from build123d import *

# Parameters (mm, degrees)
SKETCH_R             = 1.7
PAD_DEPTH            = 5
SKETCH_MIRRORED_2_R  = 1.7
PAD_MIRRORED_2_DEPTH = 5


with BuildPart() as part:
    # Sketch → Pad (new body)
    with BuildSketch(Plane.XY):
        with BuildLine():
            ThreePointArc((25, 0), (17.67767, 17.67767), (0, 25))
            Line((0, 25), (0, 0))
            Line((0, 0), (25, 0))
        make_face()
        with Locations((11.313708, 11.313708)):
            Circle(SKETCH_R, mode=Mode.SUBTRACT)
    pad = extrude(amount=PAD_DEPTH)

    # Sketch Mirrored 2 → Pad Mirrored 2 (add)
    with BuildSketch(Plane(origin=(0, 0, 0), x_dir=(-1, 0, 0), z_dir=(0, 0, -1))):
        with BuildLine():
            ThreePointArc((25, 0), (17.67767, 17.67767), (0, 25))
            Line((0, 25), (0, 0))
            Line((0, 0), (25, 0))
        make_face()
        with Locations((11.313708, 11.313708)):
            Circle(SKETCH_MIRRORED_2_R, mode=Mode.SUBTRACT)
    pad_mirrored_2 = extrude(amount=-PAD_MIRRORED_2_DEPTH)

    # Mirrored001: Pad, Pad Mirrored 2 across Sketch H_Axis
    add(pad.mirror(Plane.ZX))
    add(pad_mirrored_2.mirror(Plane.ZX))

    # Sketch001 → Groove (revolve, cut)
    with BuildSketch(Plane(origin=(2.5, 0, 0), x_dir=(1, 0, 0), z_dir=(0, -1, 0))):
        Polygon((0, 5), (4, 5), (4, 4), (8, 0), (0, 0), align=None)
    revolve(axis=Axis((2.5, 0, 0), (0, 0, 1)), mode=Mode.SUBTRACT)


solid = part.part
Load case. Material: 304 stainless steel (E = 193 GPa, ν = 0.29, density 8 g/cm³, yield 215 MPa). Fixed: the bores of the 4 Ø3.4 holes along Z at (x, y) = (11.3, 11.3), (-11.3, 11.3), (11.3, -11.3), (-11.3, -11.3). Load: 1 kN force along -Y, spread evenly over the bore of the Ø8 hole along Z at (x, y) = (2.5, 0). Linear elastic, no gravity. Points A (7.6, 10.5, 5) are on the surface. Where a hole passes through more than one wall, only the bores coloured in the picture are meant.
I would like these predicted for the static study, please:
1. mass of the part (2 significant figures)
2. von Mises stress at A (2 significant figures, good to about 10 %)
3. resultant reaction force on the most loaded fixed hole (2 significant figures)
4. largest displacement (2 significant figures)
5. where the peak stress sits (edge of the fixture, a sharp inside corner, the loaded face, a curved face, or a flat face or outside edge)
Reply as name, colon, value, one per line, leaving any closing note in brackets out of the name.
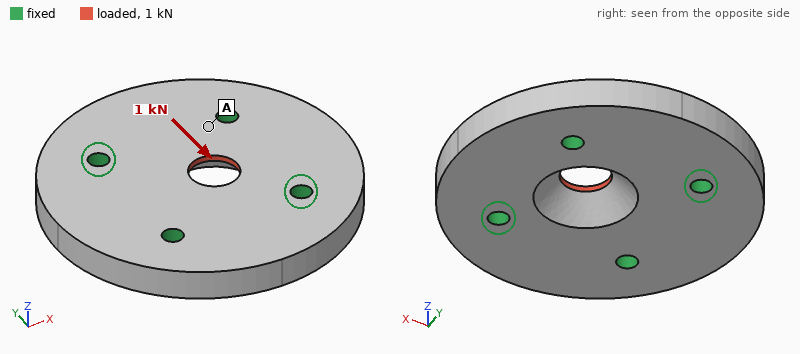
mass of the part: 73 g
von Mises stress at A: 7.8 MPa
resultant reaction force on the most loaded fixed hole: 300 N
largest displacement: 1.4 µm
where the peak stress sits: the loaded face
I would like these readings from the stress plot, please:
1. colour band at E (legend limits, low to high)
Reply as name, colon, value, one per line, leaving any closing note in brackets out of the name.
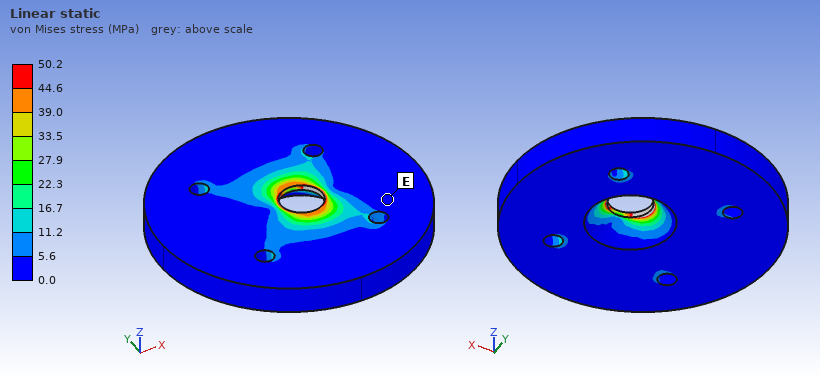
colour band at E: 0.0 to 5.6 MPa
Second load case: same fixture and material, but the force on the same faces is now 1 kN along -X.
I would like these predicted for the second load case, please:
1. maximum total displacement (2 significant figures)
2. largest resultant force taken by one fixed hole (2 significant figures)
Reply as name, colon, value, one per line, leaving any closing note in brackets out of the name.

maximum total displacement: 1.4 µm
largest resultant force taken by one fixed hole: 290 N
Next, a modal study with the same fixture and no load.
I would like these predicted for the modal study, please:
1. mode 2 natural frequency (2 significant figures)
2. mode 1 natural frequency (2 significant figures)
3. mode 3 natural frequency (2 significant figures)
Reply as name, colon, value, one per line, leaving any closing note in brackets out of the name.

mode 2 natural frequency: 21 kHz
mode 1 natural frequency: 19 kHz
mode 3 natural frequency: 21 kHz
